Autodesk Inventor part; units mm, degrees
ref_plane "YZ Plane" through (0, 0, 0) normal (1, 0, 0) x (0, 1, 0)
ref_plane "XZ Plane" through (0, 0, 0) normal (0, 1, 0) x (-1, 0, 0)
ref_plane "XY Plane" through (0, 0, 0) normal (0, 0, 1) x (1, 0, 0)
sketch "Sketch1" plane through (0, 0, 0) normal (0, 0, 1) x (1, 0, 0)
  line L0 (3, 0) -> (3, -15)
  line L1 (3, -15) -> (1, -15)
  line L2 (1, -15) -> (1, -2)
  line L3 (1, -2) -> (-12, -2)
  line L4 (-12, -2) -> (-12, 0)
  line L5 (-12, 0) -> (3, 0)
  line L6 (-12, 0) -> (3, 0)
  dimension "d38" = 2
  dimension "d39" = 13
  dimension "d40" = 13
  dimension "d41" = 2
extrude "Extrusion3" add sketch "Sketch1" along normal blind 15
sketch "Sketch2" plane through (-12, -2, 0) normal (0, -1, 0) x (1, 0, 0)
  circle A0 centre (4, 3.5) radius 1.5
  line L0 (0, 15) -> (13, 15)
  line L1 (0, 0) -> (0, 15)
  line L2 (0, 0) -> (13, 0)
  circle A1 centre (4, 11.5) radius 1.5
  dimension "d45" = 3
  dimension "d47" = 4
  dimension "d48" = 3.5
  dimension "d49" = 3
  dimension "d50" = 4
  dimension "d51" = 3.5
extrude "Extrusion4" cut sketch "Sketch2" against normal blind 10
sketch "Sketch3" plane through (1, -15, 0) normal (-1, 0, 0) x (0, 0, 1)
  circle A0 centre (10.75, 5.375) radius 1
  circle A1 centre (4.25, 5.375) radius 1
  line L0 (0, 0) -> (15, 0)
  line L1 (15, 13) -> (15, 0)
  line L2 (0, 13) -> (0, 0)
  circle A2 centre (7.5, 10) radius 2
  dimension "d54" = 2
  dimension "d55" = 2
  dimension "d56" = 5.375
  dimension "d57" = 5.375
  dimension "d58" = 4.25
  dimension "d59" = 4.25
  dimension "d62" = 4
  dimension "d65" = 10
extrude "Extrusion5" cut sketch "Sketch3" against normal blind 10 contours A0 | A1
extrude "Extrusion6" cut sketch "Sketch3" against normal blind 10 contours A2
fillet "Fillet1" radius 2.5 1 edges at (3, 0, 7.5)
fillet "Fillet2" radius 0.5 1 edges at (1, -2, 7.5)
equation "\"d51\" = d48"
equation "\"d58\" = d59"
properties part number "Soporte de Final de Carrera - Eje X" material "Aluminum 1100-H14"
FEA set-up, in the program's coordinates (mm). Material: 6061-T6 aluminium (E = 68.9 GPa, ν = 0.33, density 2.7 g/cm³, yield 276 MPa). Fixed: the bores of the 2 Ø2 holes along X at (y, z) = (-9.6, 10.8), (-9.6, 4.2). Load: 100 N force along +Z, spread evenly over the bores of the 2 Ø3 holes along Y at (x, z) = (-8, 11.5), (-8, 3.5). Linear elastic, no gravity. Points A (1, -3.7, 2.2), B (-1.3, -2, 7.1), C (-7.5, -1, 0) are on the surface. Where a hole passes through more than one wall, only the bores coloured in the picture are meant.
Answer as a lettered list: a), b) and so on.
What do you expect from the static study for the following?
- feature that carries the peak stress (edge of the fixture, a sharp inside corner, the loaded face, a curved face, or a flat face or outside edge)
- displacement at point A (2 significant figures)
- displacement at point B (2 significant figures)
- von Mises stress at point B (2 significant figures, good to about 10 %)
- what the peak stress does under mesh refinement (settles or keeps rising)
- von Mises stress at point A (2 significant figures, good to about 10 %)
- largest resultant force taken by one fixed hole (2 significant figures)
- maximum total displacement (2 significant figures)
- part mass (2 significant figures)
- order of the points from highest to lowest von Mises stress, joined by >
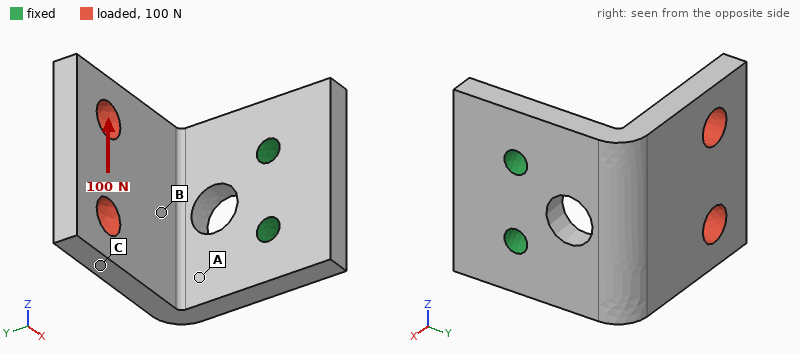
a) edge of the fixture
b) 18 µm
c) 20 µm
d) 27 MPa
e) keeps rising
f) 58 MPa
g) 150 N
h) 86 µm
i) 2.0 g
j) A > B > C
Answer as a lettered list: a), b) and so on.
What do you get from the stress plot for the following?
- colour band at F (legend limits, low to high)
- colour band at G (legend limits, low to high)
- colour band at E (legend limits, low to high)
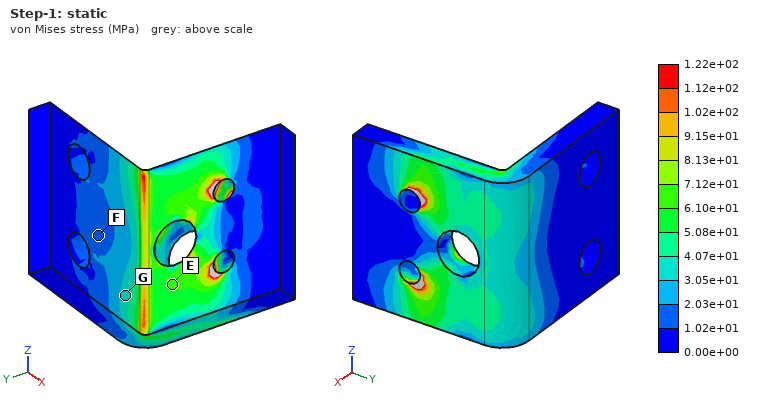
a) 1.02e+01 to 2.03e+01 MPa
b) 3.05e+01 to 4.07e+01 MPa
c) 6.10e+01 to 7.12e+01 MPa
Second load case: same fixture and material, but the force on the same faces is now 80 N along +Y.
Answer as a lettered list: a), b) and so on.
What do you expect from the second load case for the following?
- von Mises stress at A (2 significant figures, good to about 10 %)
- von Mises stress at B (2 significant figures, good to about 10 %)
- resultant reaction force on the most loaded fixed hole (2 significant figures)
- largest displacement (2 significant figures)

a) 97 MPa
b) 47 MPa
c) 41 N
d) 0.22 mm
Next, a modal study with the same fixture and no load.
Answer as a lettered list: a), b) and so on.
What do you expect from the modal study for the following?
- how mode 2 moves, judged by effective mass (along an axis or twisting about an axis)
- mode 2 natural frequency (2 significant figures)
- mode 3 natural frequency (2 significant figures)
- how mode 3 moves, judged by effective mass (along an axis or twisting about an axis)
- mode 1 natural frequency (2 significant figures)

a) along Z
b) 7300 Hz
c) 13 kHz
d) along X
e) 4200 Hz
